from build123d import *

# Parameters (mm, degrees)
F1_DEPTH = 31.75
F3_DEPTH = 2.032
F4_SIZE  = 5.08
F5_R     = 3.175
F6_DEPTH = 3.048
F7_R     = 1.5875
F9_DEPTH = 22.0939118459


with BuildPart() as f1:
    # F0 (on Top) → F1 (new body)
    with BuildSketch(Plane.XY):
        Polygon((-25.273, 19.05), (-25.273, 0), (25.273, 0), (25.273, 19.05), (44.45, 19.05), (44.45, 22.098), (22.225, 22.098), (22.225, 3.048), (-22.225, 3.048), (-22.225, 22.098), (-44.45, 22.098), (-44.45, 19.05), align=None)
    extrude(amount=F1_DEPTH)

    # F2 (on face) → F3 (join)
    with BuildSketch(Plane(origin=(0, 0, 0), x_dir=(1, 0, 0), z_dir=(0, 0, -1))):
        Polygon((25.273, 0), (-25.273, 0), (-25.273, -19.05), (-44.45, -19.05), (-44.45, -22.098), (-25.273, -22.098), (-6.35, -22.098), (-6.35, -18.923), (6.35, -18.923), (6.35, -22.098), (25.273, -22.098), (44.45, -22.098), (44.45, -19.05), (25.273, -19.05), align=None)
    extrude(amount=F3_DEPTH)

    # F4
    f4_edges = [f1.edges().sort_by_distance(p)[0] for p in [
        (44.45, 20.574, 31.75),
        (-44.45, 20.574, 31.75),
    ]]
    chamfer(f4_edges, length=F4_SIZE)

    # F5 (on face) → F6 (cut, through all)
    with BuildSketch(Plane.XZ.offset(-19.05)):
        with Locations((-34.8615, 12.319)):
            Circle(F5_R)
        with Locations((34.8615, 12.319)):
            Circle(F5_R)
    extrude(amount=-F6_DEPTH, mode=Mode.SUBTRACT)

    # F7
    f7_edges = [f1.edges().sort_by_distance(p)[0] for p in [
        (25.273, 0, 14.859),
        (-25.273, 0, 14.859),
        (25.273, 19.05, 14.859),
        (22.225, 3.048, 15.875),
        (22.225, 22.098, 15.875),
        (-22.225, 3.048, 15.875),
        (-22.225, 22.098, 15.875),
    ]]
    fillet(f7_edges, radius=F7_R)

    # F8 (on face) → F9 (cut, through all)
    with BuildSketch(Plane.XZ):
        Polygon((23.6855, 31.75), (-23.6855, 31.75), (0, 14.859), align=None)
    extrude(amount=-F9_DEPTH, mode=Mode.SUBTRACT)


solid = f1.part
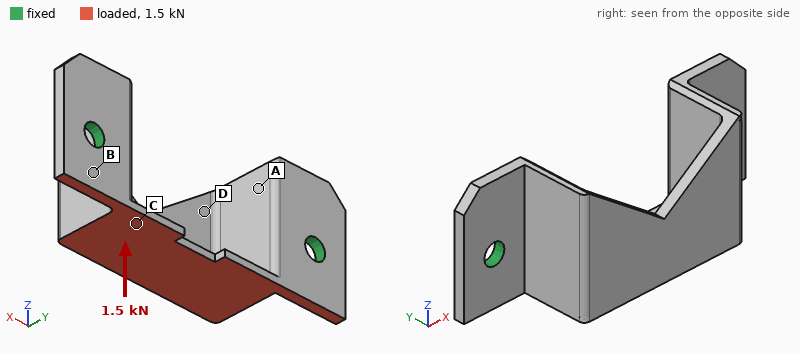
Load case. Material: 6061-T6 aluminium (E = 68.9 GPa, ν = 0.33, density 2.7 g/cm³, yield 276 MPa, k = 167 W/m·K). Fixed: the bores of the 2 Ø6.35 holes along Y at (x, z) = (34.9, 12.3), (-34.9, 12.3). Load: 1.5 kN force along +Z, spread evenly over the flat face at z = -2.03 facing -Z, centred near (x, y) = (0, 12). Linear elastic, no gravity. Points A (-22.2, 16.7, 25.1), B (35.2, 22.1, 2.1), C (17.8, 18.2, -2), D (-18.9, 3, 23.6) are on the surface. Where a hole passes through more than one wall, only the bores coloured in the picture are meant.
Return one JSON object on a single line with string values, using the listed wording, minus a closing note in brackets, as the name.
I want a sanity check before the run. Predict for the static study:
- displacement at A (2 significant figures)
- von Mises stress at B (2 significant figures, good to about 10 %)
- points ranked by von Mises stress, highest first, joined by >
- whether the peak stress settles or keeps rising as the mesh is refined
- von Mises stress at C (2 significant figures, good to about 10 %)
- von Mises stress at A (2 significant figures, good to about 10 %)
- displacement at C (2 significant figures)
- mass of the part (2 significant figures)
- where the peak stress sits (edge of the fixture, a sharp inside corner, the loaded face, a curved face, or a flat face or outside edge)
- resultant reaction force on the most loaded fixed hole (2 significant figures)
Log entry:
{"displacement at A": "0.080 mm", "von Mises stress at B": "51 MPa", "points ranked by von Mises stress, highest first, joined by >": "C > B > A > D", "whether the peak stress settles or keeps rising as the mesh is refined": "keeps rising", "von Mises stress at C": "70 MPa", "von Mises stress at A": "29 MPa", "displacement at C": "0.098 mm", "mass of the part": "36 g", "where the peak stress sits": "edge of the fixture", "resultant reaction force on the most loaded fixed hole": "800 N"}
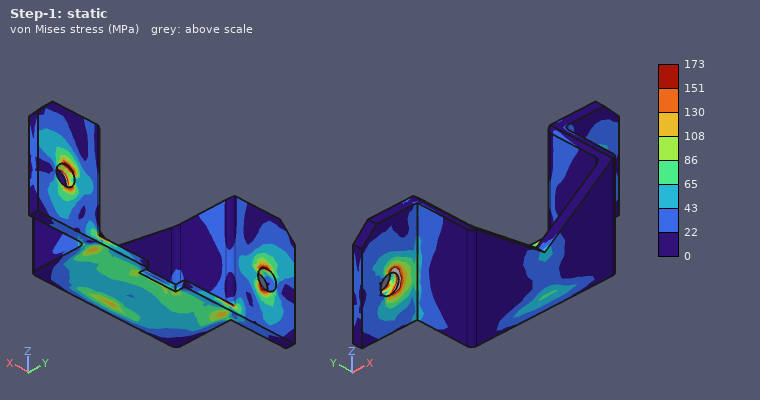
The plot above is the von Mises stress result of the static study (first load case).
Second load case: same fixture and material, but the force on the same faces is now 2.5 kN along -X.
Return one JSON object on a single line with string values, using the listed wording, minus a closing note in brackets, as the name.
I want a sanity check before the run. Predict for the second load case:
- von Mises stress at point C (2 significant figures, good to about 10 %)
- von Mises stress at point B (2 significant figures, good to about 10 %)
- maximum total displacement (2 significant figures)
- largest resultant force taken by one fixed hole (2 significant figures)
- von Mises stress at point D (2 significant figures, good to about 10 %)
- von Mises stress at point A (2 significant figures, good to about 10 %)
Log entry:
{"von Mises stress at point C": "26 MPa", "von Mises stress at point B": "32 MPa", "maximum total displacement": "60 µm", "largest resultant force taken by one fixed hole": "1.3 kN", "von Mises stress at point D": "31 MPa", "von Mises stress at point A": "24 MPa"}
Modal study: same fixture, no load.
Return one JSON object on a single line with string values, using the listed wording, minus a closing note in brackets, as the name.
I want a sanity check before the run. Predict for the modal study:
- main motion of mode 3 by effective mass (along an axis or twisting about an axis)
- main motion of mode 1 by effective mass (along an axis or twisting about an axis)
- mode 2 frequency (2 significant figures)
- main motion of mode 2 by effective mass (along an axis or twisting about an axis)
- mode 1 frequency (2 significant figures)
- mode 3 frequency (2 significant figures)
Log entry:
{"main motion of mode 3 by effective mass": "along Y", "main motion of mode 1 by effective mass": "along Z", "mode 2 frequency": "3600 Hz", "main motion of mode 2 by effective mass": "along X", "mode 1 frequency": "2700 Hz", "mode 3 frequency": "6500 Hz"}
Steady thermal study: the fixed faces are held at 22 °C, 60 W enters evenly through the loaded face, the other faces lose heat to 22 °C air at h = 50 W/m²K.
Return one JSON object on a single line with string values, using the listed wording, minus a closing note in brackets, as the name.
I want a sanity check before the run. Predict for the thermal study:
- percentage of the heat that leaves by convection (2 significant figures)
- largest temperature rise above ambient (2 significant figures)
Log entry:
{"percentage of the heat that leaves by convection": "18 %", "largest temperature rise above ambient": "57 K"}
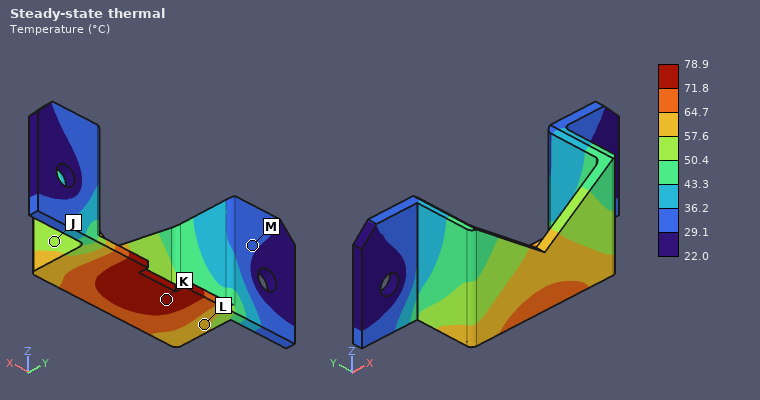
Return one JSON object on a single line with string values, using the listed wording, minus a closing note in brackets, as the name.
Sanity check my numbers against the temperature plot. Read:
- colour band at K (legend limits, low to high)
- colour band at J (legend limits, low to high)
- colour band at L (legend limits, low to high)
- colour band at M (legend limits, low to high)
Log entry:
{"colour band at K": "71.8 to 78.9 °C", "colour band at J": "50.4 to 57.6 °C", "colour band at L": "57.6 to 64.7 °C", "colour band at M": "29.1 to 36.2 °C"}
